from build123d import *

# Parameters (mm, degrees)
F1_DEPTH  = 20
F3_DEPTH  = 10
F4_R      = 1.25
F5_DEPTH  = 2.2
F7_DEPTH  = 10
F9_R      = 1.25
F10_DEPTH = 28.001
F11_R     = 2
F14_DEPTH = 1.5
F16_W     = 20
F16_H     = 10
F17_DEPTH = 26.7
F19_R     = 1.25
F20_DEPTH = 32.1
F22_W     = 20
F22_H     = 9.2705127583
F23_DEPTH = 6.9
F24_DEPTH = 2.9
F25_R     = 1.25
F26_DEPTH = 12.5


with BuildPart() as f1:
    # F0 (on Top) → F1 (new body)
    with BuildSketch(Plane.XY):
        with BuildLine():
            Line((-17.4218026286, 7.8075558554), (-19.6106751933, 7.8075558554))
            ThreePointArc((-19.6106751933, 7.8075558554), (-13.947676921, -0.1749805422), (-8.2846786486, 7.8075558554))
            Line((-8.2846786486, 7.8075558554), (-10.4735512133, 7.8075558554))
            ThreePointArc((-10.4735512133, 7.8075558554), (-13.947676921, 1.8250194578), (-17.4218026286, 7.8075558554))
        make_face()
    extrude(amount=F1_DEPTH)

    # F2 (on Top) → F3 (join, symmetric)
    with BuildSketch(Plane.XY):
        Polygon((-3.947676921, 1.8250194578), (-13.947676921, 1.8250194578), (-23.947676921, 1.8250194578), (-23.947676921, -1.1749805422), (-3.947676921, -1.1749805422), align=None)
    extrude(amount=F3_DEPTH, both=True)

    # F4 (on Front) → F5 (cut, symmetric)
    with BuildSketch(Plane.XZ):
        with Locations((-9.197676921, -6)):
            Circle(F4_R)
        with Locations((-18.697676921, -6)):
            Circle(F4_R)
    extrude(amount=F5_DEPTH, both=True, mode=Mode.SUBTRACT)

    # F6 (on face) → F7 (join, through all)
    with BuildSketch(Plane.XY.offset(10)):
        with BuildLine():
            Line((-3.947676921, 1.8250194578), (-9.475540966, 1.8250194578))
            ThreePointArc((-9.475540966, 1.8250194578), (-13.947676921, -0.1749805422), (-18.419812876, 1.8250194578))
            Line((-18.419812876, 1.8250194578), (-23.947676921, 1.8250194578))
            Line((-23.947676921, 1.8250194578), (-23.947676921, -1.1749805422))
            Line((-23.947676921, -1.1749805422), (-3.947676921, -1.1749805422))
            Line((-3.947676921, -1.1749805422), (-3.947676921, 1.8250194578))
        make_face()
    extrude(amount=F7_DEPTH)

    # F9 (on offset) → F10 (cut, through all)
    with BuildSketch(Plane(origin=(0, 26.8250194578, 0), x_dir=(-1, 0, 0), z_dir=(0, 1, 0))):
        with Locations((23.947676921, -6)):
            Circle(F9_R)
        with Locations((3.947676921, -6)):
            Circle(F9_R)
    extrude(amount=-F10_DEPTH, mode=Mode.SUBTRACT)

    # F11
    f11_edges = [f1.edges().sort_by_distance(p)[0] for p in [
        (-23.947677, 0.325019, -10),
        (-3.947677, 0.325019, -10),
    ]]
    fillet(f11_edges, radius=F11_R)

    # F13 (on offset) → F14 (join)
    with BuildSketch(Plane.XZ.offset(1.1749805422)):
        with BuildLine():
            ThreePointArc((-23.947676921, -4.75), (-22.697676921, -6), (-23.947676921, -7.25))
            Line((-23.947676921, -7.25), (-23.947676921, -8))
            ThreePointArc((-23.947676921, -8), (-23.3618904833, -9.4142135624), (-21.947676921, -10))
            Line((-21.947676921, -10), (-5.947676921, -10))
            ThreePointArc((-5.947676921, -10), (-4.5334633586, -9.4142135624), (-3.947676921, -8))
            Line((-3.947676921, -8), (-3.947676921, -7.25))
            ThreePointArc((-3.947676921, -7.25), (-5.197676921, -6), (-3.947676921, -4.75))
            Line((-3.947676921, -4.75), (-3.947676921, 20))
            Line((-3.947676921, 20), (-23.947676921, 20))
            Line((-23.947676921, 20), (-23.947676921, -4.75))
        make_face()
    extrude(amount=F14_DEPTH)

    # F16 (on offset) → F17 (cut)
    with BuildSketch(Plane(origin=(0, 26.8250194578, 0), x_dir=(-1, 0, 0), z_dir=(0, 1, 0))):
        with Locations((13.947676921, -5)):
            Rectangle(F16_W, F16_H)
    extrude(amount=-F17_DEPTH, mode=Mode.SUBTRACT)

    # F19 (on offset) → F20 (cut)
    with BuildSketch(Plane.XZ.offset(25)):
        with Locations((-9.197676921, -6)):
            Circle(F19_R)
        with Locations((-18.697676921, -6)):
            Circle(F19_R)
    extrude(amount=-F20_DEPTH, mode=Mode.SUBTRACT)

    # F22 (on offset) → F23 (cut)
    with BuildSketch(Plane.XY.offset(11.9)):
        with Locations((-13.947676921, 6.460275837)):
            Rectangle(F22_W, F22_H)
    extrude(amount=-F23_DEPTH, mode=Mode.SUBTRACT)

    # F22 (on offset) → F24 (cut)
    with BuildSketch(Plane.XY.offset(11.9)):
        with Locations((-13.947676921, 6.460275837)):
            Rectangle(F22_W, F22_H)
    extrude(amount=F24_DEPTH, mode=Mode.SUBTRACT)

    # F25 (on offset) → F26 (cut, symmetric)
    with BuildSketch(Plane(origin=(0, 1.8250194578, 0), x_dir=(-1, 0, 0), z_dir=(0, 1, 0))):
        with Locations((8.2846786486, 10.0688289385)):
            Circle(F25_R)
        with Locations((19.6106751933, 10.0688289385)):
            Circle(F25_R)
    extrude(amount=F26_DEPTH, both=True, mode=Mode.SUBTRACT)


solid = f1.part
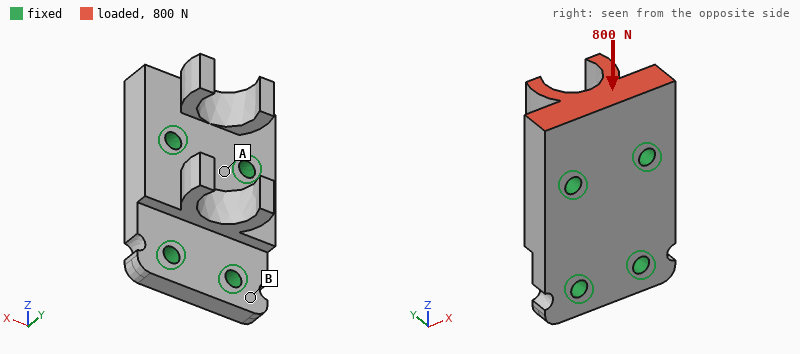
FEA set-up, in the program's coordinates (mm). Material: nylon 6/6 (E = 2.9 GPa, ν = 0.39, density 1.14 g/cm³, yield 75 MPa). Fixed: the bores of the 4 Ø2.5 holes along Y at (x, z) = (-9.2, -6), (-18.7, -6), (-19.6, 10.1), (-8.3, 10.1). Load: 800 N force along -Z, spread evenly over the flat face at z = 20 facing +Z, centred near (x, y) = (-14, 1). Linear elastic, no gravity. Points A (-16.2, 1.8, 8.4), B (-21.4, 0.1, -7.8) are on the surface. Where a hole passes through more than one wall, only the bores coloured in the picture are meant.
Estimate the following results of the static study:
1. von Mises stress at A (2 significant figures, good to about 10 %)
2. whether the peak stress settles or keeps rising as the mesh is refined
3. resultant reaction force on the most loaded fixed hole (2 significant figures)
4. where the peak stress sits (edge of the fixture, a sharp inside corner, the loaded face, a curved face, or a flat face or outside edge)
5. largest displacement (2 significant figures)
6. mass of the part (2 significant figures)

8.2 MPa
keeps rising
380 N
edge of the fixture
0.28 mm
2.9 g
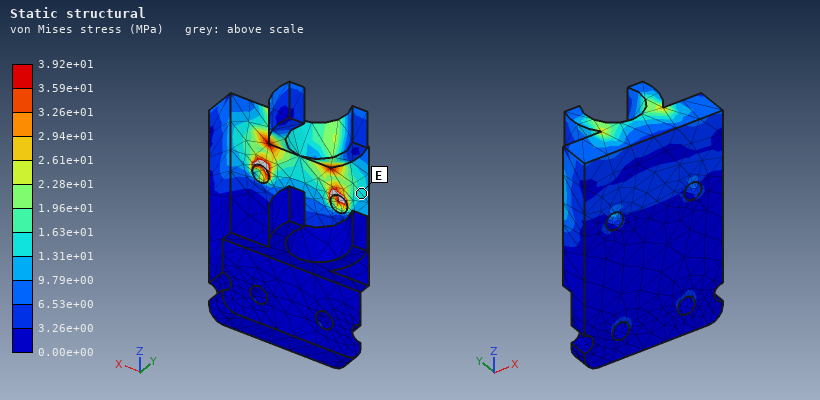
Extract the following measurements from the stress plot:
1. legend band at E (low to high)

1.31e+01 to 1.63e+01 MPa
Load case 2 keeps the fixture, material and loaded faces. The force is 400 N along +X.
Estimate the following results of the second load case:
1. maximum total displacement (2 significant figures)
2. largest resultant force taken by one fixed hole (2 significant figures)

0.30 mm
330 N
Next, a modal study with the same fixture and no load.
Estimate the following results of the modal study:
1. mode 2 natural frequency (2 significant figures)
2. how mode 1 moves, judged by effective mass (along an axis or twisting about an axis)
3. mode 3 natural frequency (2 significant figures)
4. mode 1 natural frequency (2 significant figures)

9800 Hz
along Y
11 kHz
8200 Hz
